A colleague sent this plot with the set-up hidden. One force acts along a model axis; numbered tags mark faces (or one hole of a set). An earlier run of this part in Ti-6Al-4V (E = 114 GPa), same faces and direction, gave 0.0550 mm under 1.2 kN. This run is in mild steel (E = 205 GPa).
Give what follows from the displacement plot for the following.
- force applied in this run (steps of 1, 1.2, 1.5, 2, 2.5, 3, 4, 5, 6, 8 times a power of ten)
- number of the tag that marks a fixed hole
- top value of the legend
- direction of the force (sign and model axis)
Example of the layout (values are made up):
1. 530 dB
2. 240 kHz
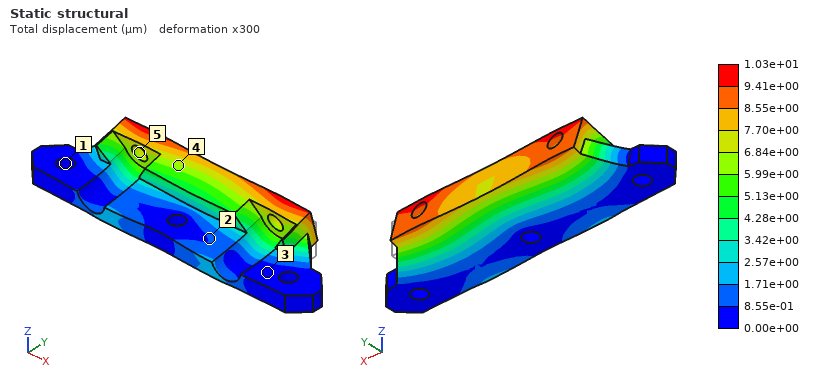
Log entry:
1. 400 N
2. 1
3. 1.03e+01 µm
4. +Z
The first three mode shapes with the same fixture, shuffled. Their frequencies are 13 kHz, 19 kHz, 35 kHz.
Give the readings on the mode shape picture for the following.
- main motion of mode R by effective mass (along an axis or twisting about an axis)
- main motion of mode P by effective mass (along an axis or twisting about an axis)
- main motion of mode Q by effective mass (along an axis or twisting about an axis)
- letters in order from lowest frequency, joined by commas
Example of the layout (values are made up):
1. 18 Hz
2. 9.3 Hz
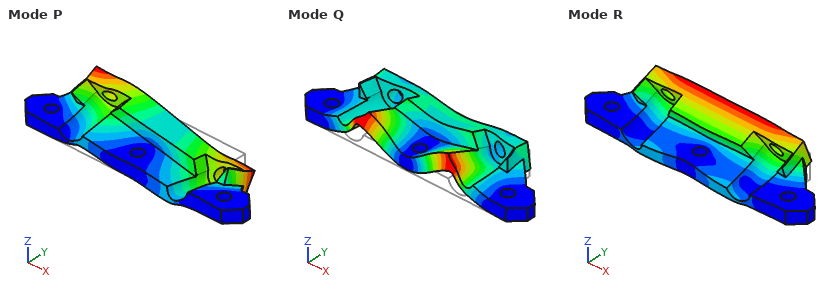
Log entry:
1. along Z
2. twisting about Y
3. along Z
4. R, P, Q
